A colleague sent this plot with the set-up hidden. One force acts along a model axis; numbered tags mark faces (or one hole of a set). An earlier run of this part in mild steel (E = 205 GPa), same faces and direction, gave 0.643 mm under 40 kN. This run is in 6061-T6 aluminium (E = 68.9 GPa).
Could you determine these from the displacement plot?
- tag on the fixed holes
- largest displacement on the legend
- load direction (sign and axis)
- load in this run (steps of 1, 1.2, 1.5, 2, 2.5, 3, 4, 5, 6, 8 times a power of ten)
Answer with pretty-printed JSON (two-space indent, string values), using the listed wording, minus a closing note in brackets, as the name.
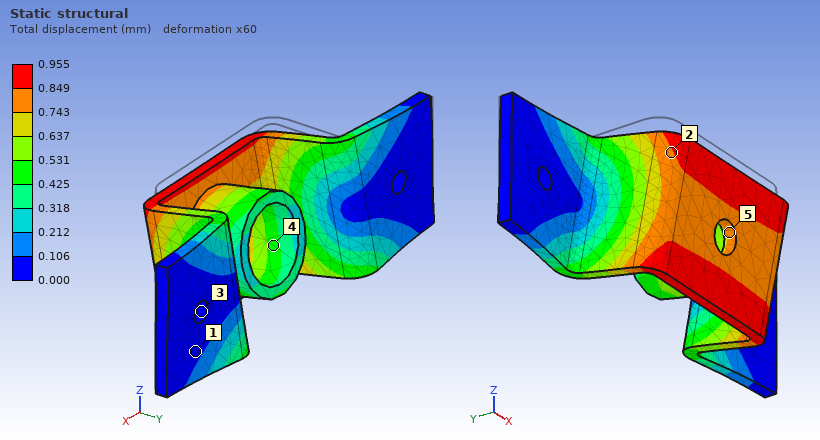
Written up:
{
  "tag on the fixed holes": "3",
  "largest displacement on the legend": "0.955 mm",
  "load direction": "-Z",
  "load in this run": "20 kN"
}
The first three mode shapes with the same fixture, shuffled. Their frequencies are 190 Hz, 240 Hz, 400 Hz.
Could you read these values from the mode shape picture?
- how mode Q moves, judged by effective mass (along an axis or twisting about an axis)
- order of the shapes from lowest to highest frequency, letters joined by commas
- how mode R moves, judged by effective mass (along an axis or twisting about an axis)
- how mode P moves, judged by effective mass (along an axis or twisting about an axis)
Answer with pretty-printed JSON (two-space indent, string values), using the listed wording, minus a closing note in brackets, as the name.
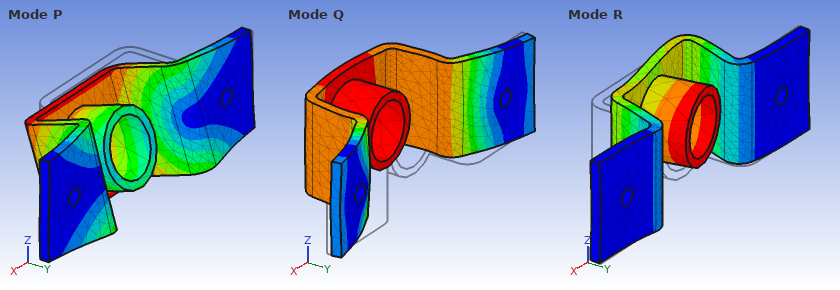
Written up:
{
  "how mode Q moves, judged by effective mass": "along Y",
  "order of the shapes from lowest to highest frequency, letters joined by commas": "P, R, Q",
  "how mode R moves, judged by effective mass": "along X",
  "how mode P moves, judged by effective mass": "along Z"
}
